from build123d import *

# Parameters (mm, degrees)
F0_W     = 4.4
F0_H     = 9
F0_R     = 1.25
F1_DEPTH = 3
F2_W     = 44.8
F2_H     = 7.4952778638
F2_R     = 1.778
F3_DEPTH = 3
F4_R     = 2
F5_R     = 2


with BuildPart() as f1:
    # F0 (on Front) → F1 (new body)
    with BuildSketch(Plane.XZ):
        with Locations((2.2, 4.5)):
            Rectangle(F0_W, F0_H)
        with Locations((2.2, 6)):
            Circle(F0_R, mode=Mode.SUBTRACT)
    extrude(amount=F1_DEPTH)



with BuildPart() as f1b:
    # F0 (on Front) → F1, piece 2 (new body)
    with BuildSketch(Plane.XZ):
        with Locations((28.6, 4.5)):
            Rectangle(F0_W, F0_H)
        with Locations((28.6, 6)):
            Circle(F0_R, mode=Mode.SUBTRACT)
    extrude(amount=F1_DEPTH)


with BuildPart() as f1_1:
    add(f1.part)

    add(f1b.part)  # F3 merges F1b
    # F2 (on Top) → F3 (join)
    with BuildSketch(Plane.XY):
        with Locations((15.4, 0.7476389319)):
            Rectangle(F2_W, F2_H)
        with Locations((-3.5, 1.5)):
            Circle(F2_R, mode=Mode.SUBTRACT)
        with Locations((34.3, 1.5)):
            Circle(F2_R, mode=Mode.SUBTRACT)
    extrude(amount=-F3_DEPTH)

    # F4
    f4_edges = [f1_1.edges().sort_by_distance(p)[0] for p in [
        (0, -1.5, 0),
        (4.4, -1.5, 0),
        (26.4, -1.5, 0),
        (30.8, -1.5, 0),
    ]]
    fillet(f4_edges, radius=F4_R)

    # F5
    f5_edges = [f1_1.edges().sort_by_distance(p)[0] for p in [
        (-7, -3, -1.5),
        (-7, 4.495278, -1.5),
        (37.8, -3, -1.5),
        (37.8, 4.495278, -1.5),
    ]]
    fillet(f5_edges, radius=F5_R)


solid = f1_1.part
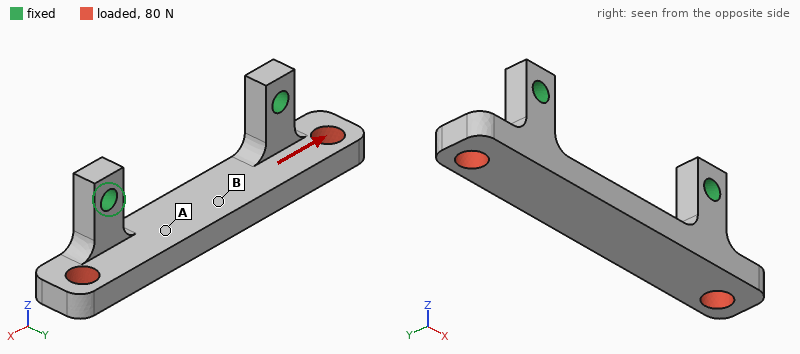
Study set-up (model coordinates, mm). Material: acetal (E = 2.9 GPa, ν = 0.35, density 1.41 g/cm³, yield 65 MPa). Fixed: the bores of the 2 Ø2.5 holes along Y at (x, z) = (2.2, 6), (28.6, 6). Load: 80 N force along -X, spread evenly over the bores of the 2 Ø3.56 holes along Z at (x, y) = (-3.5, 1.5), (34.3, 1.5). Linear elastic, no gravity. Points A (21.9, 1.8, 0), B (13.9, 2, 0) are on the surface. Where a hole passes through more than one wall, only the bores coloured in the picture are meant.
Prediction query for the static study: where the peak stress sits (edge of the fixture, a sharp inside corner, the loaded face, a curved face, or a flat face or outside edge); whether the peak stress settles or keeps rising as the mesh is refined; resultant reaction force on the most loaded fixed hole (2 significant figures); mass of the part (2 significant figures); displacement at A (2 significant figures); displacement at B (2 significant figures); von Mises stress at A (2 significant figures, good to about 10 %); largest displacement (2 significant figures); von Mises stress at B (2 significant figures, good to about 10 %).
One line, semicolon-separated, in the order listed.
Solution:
edge of the fixture; keeps rising; 42 N; 1.6 g; 0.071 mm; 0.071 mm; 4.3 MPa; 0.12 mm; 1.7 MPa
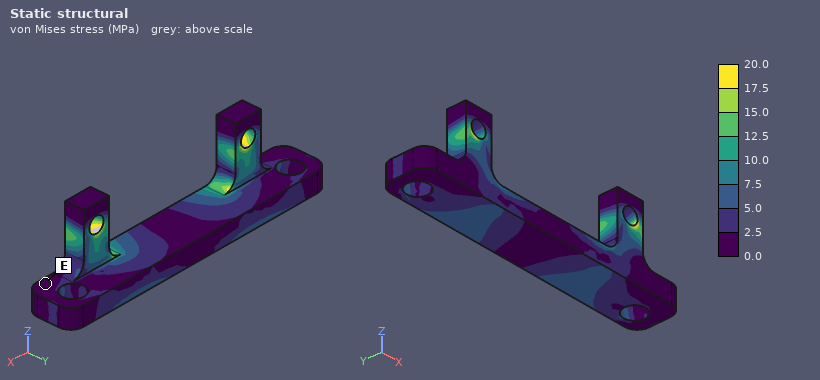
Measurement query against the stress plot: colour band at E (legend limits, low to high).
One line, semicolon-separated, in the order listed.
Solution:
0.0 to 2.5 MPa
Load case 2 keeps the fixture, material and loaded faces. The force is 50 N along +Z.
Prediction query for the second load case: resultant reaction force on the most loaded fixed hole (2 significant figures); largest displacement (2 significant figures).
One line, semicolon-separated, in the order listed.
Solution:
31 N; 0.21 mm
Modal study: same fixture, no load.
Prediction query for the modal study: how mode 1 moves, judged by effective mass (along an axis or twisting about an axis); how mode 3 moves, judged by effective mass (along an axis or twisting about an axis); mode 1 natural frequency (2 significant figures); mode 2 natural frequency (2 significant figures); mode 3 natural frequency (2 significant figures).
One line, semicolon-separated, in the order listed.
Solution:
along Y; along X; 2600 Hz; 3700 Hz; 4400 Hz
